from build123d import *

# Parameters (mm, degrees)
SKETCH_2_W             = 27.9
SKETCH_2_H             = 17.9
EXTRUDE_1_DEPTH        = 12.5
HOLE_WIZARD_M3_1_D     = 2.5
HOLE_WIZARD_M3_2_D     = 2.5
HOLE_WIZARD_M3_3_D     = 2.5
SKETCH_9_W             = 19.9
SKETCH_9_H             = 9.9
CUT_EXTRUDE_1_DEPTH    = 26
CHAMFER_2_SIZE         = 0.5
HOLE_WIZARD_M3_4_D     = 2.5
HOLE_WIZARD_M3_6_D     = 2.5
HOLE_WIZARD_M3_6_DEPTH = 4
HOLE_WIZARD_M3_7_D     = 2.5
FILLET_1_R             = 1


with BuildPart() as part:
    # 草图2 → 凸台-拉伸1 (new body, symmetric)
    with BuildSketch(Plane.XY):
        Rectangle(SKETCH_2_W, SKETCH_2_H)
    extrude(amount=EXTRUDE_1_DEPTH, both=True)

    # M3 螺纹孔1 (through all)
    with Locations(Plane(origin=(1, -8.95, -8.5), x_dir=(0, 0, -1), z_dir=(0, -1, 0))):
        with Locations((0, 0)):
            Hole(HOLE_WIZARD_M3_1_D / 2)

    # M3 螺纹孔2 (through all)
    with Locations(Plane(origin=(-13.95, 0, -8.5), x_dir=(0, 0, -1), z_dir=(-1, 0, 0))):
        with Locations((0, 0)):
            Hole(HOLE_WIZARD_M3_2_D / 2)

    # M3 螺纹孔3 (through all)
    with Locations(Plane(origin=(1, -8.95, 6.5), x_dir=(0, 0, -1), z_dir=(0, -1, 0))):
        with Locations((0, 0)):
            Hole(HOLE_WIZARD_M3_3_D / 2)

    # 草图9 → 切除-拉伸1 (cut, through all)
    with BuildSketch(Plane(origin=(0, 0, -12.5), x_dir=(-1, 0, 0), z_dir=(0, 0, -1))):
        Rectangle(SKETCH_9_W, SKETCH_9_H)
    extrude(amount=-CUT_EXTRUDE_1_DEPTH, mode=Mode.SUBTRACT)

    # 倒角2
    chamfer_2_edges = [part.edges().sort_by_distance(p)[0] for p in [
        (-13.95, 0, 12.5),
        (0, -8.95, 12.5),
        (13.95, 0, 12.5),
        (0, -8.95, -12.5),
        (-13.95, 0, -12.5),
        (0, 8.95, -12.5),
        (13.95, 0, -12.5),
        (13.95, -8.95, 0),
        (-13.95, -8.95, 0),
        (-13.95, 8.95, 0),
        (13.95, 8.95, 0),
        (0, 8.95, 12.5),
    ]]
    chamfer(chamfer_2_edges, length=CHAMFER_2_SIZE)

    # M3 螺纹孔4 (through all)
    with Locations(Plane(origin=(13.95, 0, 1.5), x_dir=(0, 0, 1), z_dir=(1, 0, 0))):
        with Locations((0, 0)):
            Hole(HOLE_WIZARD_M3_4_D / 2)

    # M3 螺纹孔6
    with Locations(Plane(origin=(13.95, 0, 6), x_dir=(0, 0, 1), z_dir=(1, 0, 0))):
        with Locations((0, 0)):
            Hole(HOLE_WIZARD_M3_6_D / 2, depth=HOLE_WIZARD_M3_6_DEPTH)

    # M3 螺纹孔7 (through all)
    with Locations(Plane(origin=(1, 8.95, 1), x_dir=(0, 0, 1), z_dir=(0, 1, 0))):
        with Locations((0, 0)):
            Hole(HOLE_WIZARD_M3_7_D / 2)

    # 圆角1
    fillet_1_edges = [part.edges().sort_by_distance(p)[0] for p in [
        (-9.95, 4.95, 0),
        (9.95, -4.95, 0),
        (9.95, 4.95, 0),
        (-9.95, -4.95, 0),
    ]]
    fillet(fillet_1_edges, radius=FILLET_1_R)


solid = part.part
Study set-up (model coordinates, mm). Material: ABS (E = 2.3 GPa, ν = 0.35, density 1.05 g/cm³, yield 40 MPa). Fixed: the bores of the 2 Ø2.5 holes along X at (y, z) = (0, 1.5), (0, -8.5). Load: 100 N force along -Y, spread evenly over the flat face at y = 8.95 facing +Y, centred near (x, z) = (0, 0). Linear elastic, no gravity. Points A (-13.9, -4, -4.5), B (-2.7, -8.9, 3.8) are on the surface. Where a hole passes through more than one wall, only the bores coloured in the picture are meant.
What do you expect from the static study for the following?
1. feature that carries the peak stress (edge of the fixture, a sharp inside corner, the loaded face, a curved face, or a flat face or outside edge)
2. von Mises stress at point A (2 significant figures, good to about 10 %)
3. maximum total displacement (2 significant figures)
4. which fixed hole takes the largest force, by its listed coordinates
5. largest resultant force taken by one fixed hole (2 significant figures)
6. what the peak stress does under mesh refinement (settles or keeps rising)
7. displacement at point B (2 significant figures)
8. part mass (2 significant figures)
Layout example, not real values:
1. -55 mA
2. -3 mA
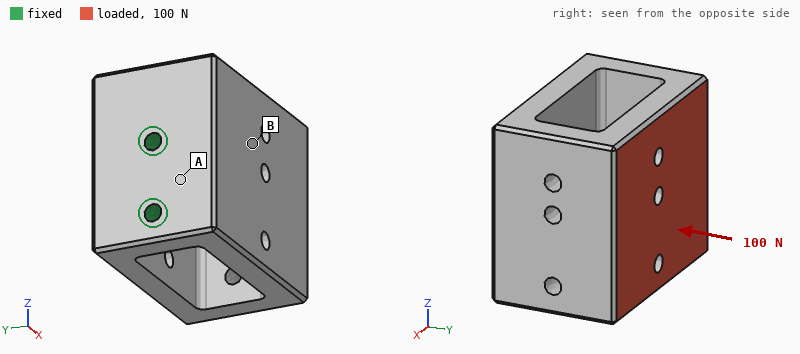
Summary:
1. edge of the fixture
2. 4.8 MPa
3. 0.39 mm
4. (0, 1.5)
5. 80 N
6. keeps rising
7. 0.16 mm
8. 7.7 g
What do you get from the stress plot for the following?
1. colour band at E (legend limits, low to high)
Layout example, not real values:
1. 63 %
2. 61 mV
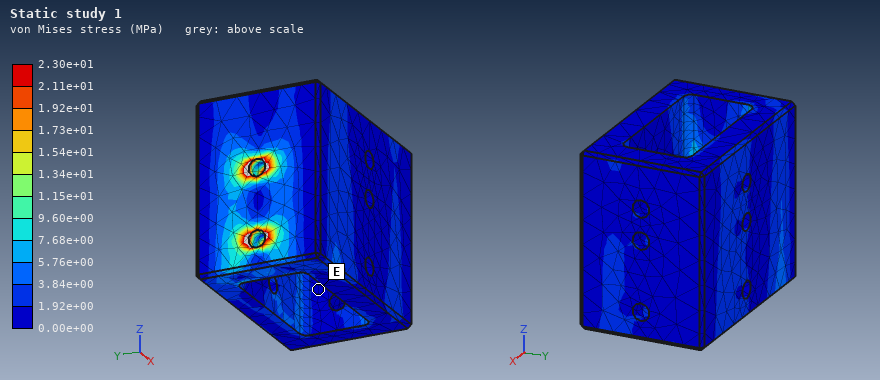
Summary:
1. 0.00e+00 to 1.92e+00 MPa
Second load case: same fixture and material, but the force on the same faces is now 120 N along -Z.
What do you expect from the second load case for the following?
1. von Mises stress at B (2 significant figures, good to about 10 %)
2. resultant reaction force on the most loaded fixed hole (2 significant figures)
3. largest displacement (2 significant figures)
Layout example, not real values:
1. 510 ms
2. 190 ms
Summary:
1. 1.2 MPa
2. 150 N
3. 0.20 mm
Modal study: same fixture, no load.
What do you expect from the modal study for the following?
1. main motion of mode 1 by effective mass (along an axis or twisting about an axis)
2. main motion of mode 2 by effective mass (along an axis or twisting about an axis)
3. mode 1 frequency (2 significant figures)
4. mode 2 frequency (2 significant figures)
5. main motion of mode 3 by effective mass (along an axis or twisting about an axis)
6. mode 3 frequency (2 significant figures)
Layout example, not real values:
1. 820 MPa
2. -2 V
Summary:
1. along Y
2. along Z
3. 1000 Hz
4. 1800 Hz
5. twisting about X
6. 3100 Hz
